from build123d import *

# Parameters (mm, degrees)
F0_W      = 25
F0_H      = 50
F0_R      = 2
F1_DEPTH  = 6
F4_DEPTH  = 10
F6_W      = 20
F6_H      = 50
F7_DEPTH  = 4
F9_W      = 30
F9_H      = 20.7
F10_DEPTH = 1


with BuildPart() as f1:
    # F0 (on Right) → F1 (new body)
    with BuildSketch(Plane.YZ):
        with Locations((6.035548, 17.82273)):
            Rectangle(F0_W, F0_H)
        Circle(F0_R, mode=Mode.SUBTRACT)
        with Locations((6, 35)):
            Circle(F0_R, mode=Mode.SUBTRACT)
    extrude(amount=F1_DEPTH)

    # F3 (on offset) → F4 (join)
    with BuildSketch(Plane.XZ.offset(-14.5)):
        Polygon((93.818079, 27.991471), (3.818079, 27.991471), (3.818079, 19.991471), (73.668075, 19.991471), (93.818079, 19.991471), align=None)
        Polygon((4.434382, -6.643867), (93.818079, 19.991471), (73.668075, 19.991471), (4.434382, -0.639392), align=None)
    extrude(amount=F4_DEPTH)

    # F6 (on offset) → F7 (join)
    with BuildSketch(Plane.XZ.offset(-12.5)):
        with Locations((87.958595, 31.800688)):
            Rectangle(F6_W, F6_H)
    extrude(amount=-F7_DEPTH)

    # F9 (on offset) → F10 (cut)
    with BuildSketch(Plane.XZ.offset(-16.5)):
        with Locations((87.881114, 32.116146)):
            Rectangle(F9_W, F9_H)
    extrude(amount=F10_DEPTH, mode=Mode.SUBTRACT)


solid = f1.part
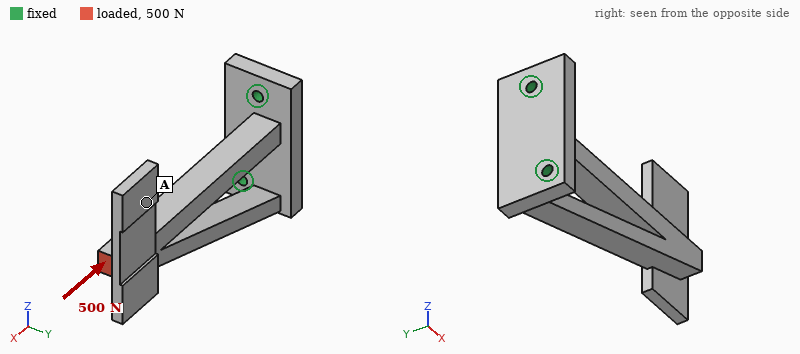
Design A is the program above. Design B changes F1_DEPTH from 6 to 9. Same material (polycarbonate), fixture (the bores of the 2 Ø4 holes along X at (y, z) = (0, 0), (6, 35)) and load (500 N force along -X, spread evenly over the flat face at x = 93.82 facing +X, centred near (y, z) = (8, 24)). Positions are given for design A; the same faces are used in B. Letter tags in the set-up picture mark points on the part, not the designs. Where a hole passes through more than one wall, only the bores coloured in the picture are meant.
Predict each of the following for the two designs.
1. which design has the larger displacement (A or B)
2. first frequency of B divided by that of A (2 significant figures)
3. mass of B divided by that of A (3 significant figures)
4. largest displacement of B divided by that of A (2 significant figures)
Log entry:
A
1.2
1.15
0.86
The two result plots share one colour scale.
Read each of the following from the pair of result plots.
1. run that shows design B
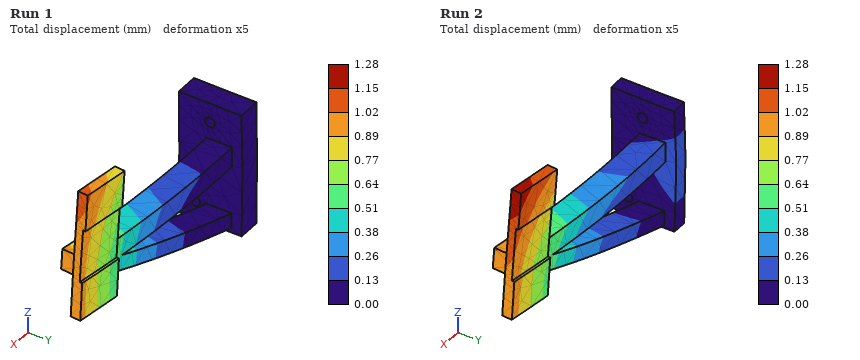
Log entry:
Run 1
